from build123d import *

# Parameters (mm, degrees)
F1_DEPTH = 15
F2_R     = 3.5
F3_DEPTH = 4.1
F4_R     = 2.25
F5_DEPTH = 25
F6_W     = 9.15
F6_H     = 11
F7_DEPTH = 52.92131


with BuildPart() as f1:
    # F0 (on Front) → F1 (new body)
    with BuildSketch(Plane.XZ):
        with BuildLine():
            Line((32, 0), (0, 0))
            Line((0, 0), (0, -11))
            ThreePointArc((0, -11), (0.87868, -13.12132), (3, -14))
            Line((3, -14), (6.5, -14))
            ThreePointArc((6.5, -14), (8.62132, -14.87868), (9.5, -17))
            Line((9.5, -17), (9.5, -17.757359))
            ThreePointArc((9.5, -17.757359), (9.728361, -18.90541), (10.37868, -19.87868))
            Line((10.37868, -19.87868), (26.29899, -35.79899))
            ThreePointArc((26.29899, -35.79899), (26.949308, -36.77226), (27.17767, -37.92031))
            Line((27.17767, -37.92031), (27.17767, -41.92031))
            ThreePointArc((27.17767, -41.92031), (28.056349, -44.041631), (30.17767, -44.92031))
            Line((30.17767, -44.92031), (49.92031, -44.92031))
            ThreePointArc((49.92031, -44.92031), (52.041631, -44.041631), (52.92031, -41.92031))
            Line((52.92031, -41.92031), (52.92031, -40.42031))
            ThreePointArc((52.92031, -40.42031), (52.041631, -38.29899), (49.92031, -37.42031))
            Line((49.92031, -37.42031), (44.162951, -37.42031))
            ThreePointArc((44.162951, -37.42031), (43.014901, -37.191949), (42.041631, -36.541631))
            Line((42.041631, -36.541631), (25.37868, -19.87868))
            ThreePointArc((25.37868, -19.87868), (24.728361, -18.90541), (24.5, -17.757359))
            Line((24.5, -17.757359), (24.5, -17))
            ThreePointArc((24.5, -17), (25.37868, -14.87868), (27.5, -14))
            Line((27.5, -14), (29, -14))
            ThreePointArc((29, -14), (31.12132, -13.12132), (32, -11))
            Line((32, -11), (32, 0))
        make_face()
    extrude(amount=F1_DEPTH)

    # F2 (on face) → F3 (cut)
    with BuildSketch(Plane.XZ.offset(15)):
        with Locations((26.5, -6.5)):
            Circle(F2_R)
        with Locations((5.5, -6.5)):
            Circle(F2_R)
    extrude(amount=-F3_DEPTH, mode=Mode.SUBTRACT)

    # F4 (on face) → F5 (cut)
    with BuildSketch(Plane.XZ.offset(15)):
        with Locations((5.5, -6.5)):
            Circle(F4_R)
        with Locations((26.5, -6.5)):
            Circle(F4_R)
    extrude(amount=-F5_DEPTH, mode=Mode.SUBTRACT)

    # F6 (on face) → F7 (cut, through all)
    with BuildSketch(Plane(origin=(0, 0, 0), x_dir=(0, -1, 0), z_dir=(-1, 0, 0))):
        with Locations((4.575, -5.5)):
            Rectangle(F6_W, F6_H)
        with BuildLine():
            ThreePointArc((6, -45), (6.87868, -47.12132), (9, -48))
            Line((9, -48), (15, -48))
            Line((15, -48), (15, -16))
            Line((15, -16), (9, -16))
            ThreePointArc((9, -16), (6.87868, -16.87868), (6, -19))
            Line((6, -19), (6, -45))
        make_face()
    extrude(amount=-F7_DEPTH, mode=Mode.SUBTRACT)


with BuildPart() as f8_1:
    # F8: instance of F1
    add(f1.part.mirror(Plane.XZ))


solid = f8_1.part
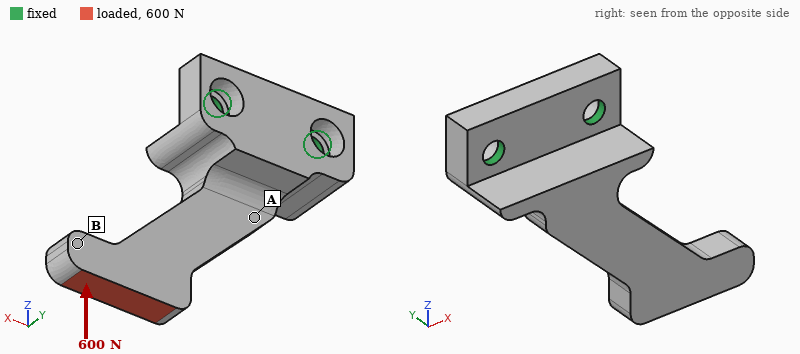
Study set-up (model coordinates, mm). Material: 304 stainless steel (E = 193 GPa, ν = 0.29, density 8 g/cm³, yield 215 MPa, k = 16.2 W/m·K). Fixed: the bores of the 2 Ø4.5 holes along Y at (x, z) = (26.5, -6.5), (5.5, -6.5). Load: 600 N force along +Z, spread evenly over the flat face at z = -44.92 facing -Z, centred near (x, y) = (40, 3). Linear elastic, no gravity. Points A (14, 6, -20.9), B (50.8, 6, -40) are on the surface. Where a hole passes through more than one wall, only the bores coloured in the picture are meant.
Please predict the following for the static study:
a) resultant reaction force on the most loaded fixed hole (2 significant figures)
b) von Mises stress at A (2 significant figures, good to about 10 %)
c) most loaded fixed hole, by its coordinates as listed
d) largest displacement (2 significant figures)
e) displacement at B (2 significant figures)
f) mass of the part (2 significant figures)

990 N
67 MPa
(26.5, -6.5)
0.13 mm
0.12 mm
53 g
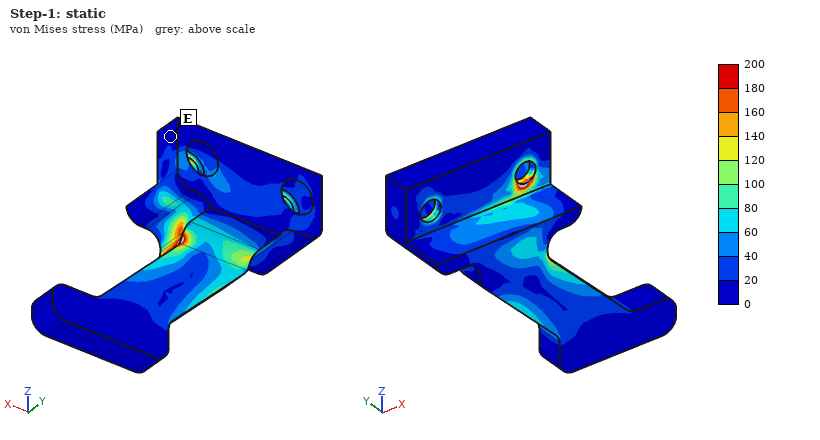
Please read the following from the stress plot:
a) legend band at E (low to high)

0 to 20 MPa
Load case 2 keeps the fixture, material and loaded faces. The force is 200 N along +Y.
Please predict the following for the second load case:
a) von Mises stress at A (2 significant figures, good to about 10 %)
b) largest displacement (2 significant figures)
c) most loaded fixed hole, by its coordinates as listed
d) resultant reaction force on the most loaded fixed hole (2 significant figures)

60 MPa
0.21 mm
(26.5, -6.5)
320 N
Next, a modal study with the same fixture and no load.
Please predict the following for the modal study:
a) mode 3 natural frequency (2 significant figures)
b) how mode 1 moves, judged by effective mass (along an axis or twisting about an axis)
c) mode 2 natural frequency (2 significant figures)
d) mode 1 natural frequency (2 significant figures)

6100 Hz
along Y
3600 Hz
1600 Hz
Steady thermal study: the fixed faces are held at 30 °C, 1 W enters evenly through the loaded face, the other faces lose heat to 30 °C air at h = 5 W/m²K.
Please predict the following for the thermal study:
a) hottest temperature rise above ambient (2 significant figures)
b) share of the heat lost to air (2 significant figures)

36 K
20 %
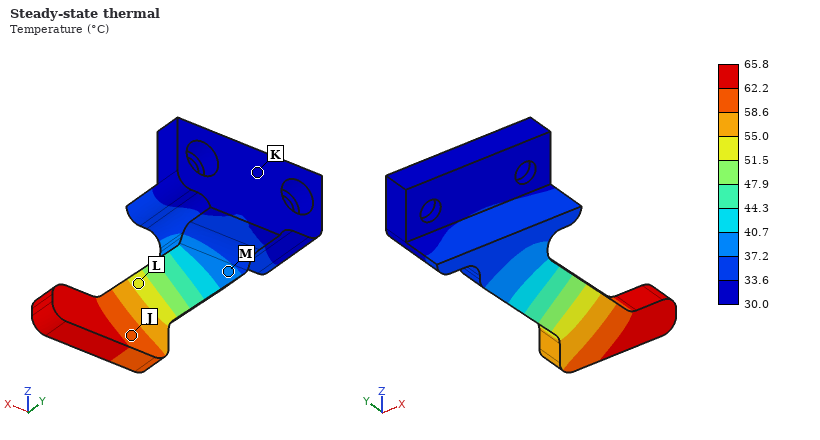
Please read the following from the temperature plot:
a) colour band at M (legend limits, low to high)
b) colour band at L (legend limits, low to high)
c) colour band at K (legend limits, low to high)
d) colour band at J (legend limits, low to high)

37.2 to 40.7 °C
51.5 to 55.0 °C
30.0 to 33.6 °C
58.6 to 62.2 °C
